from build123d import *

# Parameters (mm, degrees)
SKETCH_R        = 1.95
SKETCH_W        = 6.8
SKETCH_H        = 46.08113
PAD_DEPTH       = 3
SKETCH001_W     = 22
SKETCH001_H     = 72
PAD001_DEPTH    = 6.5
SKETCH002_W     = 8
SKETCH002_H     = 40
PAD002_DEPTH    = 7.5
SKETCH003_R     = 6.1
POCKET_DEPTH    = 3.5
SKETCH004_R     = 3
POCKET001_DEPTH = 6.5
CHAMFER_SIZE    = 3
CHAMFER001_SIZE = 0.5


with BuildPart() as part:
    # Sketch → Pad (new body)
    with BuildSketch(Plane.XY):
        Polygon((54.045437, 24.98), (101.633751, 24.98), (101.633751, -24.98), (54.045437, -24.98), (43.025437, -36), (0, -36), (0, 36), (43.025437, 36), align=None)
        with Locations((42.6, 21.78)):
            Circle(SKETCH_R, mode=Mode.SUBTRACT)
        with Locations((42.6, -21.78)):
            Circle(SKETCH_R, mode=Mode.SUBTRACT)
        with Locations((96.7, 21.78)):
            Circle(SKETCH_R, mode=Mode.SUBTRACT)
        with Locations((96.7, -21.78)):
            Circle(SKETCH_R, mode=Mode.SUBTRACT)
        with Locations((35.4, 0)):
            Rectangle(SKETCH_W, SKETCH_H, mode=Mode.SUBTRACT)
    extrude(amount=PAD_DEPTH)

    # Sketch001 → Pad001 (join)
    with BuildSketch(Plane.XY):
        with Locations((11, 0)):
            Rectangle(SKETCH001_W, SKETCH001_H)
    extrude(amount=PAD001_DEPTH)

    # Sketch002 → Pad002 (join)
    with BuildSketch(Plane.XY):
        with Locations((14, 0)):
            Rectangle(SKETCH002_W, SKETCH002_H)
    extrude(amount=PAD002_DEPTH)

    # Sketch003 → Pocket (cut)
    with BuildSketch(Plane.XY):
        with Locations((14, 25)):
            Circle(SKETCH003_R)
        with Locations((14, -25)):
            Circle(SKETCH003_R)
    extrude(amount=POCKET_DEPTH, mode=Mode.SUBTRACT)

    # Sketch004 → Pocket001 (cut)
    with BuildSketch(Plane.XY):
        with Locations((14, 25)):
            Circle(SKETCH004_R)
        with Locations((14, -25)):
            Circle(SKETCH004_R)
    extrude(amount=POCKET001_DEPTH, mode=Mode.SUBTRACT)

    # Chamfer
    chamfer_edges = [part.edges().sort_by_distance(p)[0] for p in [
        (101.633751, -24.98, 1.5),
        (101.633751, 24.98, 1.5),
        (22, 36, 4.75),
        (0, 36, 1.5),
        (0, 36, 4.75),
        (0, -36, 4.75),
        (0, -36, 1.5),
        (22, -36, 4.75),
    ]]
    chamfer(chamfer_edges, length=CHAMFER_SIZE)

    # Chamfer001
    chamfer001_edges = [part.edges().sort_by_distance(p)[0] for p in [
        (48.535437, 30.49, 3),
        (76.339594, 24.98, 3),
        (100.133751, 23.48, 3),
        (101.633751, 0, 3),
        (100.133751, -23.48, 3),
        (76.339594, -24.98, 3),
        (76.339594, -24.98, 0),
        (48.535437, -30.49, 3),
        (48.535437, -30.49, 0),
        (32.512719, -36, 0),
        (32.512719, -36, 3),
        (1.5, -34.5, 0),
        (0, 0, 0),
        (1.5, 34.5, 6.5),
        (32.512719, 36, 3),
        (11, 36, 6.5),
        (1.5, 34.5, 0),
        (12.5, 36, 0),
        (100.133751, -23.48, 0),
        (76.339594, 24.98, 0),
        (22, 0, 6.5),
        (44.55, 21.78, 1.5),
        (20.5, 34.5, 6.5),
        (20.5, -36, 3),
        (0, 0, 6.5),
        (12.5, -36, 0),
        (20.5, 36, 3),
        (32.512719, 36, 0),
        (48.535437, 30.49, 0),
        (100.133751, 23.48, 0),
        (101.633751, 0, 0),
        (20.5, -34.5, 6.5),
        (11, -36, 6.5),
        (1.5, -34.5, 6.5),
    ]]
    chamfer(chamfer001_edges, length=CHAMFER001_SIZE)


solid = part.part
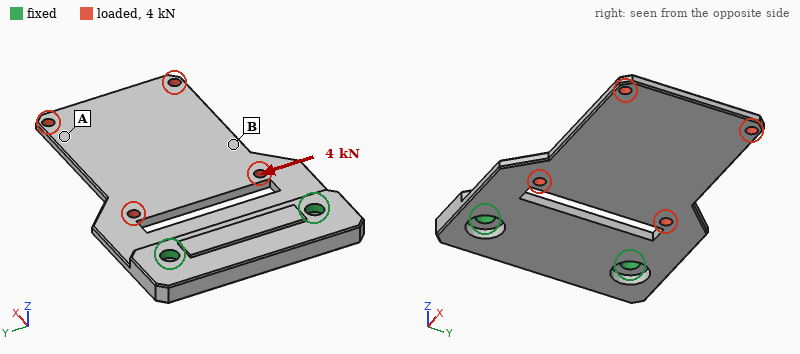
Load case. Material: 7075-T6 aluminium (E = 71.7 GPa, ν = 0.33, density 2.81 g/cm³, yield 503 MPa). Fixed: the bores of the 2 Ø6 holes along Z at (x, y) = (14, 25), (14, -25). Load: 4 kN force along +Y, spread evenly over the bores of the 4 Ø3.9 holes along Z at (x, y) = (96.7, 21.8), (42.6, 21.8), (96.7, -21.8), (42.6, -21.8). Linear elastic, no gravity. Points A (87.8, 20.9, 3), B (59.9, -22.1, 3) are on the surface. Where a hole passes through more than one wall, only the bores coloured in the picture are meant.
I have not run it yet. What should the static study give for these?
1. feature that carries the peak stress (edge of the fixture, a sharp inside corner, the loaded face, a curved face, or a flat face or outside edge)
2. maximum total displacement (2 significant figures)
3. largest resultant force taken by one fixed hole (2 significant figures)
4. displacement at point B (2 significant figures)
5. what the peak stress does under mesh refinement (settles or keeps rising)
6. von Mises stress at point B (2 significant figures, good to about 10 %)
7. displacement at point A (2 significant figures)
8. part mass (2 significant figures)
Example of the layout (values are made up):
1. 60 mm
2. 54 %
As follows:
1. a sharp inside corner
2. 0.32 mm
3. 4.5 kN
4. 0.19 mm
5. keeps rising
6. 66 MPa
7. 0.28 mm
8. 62 g
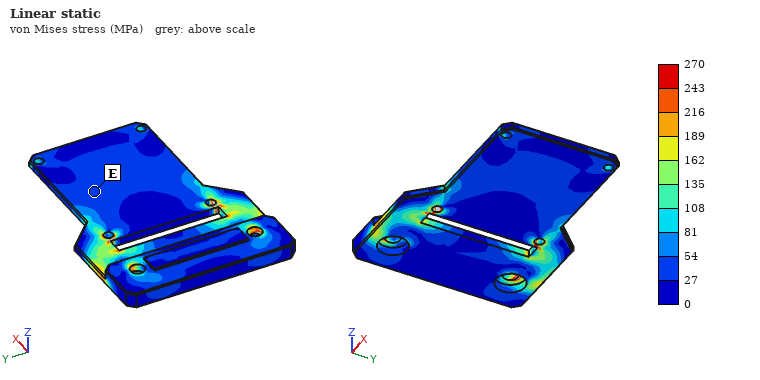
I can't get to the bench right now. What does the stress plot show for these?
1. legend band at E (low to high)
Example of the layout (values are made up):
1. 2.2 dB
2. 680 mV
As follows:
1. 27 to 54 MPa
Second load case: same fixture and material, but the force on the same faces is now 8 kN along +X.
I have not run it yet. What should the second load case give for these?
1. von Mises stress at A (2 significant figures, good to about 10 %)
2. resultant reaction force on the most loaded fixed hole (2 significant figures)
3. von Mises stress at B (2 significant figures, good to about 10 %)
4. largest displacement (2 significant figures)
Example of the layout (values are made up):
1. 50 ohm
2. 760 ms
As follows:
1. 58 MPa
2. 4.0 kN
3. 74 MPa
4. 0.60 mm
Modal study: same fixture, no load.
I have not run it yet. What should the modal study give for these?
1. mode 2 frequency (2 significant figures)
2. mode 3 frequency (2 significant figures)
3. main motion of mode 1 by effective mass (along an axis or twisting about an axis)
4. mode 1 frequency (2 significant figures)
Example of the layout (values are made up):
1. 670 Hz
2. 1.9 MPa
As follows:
1. 1400 Hz
2. 1900 Hz
3. along Z
4. 290 Hz
